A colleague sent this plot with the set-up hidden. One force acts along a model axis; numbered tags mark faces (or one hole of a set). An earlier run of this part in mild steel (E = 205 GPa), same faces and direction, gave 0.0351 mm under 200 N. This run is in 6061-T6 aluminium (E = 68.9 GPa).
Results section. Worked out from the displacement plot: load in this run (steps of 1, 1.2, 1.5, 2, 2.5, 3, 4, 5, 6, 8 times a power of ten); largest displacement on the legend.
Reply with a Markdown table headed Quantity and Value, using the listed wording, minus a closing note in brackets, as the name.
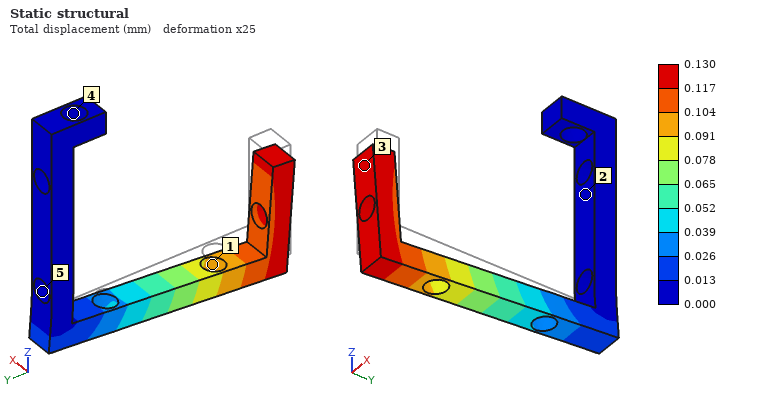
| Quantity | Value |
|---|---|
| load in this run | 250 N |
| largest displacement on the legend | 0.130 mm |
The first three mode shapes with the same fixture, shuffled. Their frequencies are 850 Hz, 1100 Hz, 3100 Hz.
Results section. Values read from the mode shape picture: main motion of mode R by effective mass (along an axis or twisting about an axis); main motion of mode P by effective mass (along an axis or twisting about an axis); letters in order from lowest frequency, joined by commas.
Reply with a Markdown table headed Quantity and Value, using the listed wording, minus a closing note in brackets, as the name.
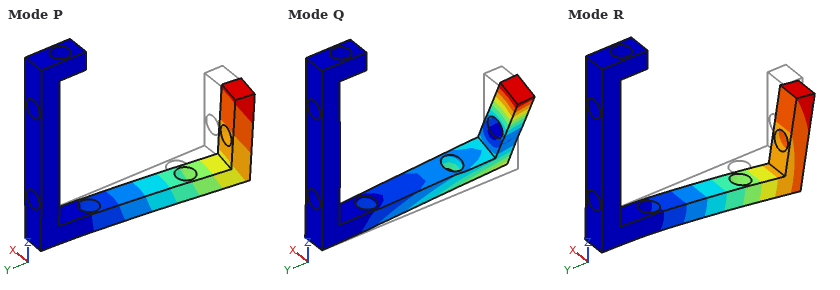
| Quantity | Value |
|---|---|
| main motion of mode R by effective mass | along Z |
| main motion of mode P by effective mass | along X |
| letters in order from lowest frequency, joined by commas | R, P, Q |
